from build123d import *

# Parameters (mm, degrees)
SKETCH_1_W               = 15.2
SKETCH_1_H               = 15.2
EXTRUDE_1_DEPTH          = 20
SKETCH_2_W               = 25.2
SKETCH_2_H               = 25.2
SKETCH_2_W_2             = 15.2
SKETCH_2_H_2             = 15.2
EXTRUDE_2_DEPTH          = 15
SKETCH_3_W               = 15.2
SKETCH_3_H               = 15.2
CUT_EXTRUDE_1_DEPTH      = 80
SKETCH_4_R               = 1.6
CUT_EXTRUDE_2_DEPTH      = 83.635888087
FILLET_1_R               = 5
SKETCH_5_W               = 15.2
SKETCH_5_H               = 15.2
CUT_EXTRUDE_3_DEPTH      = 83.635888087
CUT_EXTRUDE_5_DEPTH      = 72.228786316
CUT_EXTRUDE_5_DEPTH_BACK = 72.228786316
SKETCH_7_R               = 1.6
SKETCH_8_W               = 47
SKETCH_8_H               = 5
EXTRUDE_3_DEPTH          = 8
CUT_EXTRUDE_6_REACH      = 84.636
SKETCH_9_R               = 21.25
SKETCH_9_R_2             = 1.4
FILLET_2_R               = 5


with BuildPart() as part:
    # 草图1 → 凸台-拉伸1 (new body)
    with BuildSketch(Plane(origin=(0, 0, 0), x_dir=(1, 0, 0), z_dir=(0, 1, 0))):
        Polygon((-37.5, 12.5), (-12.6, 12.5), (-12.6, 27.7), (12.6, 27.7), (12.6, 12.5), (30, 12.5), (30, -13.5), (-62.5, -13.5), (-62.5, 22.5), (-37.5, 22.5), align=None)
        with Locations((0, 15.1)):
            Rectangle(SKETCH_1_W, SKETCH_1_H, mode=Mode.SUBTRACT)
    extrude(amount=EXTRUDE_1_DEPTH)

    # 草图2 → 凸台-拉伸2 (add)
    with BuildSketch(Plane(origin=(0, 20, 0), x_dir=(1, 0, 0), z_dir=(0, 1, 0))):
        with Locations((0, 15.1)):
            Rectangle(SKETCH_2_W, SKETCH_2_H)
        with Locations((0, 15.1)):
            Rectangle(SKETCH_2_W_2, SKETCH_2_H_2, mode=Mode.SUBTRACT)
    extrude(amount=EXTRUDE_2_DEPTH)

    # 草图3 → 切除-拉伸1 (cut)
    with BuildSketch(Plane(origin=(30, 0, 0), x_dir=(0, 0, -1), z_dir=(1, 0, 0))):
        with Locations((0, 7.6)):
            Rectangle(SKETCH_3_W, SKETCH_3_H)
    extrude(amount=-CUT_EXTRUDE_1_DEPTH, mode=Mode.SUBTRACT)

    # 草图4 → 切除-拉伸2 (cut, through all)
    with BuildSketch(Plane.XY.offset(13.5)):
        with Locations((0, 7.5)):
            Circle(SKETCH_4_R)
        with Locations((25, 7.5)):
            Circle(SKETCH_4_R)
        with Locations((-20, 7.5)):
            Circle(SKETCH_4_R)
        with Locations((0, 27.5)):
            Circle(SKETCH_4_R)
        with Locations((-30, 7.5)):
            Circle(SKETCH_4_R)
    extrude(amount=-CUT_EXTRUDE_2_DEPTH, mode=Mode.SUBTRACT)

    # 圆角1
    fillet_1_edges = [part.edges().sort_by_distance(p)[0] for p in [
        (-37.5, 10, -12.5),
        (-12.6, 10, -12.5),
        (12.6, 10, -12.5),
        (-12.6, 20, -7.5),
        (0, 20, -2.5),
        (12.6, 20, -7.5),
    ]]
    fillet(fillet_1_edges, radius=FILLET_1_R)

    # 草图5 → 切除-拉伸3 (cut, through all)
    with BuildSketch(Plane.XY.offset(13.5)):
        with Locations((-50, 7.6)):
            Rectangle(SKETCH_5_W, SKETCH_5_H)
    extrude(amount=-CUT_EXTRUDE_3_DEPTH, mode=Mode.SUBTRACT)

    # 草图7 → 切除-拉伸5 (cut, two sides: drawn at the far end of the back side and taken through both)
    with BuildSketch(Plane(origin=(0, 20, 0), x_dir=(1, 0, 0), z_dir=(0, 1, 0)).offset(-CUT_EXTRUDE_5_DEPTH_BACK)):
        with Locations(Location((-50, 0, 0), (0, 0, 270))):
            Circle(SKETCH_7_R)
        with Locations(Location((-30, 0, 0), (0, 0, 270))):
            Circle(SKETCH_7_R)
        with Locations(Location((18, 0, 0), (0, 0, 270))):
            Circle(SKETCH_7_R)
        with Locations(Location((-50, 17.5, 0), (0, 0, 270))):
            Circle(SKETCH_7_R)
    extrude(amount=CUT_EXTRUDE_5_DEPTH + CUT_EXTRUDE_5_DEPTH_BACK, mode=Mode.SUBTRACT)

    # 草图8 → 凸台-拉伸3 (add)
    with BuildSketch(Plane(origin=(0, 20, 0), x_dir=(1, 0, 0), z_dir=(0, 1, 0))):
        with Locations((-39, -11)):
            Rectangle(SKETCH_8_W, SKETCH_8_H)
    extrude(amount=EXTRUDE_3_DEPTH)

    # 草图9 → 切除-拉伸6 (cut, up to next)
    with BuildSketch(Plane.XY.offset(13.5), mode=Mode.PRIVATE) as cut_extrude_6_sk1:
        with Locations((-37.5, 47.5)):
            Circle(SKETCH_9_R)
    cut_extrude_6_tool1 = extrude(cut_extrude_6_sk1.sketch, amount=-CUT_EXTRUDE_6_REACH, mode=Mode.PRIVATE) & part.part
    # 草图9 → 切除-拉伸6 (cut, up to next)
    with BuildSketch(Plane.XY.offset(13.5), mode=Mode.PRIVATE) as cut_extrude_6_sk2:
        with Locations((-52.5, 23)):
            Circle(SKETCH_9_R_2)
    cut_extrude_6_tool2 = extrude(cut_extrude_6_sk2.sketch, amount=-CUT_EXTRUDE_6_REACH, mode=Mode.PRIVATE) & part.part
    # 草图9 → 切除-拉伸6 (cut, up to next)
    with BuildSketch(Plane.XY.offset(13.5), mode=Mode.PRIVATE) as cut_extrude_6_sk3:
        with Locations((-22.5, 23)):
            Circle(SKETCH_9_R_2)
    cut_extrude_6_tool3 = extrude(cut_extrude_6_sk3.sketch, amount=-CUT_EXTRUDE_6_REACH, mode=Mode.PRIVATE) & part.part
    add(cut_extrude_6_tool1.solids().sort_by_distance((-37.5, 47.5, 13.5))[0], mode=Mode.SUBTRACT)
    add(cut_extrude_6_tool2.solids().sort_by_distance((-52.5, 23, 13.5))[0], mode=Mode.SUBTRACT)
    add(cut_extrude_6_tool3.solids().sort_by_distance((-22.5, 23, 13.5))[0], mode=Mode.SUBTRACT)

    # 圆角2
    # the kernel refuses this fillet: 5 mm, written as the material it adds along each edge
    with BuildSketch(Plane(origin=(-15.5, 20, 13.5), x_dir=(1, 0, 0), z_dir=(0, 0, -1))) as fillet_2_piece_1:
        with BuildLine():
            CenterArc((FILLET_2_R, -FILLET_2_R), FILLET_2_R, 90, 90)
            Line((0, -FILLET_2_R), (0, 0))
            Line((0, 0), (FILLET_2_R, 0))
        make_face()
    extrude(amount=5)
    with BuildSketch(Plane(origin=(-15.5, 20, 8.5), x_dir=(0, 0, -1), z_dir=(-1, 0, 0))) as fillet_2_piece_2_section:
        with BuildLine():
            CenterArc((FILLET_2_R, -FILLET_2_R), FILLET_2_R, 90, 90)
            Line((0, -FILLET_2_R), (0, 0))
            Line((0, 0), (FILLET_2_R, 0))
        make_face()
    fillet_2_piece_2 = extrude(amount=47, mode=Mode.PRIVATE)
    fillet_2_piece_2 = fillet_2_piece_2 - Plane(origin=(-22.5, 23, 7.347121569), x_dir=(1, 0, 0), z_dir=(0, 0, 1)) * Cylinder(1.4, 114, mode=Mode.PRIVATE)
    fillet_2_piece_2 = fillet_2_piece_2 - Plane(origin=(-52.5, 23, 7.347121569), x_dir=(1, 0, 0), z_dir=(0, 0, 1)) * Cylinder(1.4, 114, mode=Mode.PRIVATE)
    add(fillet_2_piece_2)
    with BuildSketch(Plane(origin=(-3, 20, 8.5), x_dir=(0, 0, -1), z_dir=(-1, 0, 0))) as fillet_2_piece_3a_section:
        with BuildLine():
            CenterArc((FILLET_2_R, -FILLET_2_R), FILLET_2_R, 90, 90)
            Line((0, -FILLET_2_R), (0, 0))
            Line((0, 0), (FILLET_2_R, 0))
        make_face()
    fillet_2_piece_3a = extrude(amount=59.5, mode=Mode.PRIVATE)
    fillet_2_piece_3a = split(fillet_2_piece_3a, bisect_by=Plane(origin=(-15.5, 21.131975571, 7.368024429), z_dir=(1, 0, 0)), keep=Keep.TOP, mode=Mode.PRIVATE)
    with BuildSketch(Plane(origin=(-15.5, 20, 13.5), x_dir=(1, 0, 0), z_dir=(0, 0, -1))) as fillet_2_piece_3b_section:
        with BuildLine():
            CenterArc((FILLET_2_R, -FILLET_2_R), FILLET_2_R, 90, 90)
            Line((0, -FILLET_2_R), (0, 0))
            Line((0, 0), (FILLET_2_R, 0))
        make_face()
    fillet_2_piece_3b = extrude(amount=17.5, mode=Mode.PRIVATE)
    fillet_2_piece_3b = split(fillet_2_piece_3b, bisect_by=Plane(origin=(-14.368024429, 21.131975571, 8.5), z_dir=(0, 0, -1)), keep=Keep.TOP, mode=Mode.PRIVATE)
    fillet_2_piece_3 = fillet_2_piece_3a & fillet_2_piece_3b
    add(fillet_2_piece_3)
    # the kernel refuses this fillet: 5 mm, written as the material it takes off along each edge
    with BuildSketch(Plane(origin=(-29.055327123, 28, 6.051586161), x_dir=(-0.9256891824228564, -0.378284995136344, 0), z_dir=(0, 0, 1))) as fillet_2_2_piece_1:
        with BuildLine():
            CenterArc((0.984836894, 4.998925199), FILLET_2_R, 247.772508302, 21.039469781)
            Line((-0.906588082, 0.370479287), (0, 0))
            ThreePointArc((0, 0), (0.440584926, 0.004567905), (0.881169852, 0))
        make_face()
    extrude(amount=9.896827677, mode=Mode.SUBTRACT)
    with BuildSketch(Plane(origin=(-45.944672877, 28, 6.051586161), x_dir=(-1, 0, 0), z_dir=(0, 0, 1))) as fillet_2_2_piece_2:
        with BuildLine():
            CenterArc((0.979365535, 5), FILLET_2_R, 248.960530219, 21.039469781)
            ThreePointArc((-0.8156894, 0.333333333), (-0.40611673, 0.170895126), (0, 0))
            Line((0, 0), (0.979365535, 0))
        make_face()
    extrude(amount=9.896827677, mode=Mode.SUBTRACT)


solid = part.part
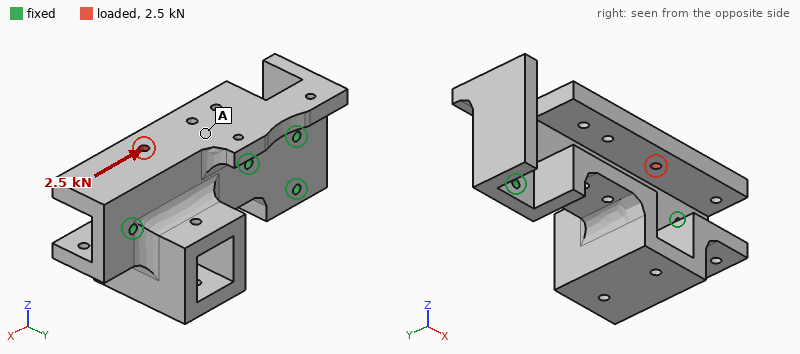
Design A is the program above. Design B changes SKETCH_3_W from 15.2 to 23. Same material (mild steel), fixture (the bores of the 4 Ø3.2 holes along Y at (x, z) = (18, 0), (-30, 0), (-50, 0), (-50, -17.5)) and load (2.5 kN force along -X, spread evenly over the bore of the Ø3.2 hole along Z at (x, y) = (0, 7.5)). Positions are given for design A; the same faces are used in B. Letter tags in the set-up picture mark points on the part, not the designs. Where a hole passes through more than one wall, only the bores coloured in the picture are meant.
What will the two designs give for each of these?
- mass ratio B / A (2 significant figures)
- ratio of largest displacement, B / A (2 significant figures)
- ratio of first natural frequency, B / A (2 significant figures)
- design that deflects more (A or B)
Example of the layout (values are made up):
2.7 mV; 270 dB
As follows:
0.81; 2.1; 0.96; B
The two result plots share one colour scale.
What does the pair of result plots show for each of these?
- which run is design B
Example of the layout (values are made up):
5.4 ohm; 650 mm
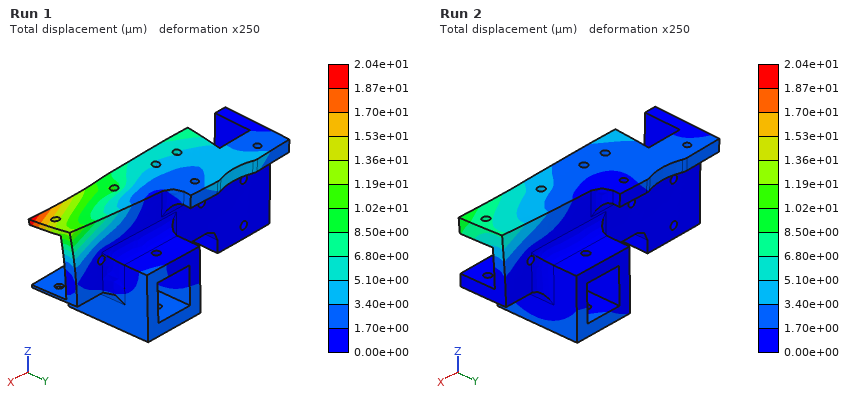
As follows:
Run 1
